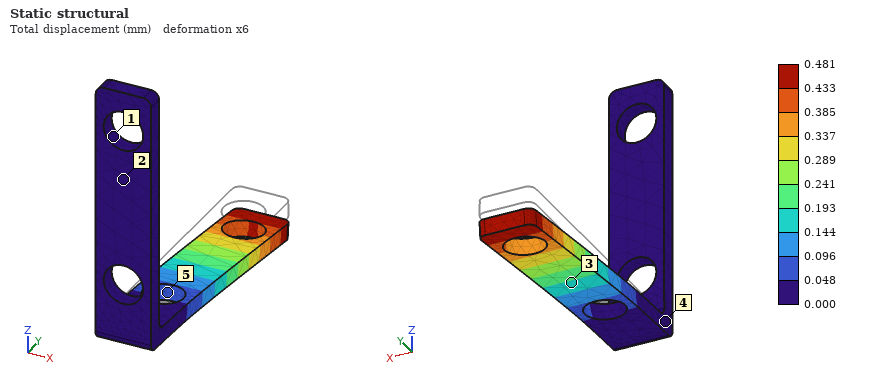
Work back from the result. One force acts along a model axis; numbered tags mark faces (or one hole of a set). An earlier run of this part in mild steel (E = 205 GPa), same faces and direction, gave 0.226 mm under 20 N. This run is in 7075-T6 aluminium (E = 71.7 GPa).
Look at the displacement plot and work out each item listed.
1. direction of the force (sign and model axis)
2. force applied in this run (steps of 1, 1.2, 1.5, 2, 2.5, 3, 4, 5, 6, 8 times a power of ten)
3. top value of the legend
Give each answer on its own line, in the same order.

-Z
15 N
0.481 mm
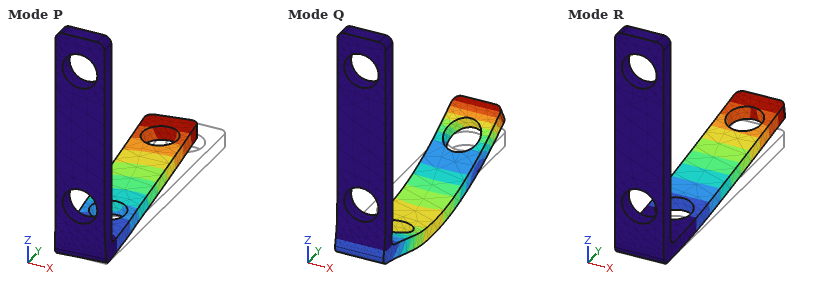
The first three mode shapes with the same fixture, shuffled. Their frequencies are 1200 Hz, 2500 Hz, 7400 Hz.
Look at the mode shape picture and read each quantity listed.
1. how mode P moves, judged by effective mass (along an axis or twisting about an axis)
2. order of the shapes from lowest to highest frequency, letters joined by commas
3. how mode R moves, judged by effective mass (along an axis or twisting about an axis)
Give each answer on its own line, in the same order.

along X
R, P, Q
along Z
